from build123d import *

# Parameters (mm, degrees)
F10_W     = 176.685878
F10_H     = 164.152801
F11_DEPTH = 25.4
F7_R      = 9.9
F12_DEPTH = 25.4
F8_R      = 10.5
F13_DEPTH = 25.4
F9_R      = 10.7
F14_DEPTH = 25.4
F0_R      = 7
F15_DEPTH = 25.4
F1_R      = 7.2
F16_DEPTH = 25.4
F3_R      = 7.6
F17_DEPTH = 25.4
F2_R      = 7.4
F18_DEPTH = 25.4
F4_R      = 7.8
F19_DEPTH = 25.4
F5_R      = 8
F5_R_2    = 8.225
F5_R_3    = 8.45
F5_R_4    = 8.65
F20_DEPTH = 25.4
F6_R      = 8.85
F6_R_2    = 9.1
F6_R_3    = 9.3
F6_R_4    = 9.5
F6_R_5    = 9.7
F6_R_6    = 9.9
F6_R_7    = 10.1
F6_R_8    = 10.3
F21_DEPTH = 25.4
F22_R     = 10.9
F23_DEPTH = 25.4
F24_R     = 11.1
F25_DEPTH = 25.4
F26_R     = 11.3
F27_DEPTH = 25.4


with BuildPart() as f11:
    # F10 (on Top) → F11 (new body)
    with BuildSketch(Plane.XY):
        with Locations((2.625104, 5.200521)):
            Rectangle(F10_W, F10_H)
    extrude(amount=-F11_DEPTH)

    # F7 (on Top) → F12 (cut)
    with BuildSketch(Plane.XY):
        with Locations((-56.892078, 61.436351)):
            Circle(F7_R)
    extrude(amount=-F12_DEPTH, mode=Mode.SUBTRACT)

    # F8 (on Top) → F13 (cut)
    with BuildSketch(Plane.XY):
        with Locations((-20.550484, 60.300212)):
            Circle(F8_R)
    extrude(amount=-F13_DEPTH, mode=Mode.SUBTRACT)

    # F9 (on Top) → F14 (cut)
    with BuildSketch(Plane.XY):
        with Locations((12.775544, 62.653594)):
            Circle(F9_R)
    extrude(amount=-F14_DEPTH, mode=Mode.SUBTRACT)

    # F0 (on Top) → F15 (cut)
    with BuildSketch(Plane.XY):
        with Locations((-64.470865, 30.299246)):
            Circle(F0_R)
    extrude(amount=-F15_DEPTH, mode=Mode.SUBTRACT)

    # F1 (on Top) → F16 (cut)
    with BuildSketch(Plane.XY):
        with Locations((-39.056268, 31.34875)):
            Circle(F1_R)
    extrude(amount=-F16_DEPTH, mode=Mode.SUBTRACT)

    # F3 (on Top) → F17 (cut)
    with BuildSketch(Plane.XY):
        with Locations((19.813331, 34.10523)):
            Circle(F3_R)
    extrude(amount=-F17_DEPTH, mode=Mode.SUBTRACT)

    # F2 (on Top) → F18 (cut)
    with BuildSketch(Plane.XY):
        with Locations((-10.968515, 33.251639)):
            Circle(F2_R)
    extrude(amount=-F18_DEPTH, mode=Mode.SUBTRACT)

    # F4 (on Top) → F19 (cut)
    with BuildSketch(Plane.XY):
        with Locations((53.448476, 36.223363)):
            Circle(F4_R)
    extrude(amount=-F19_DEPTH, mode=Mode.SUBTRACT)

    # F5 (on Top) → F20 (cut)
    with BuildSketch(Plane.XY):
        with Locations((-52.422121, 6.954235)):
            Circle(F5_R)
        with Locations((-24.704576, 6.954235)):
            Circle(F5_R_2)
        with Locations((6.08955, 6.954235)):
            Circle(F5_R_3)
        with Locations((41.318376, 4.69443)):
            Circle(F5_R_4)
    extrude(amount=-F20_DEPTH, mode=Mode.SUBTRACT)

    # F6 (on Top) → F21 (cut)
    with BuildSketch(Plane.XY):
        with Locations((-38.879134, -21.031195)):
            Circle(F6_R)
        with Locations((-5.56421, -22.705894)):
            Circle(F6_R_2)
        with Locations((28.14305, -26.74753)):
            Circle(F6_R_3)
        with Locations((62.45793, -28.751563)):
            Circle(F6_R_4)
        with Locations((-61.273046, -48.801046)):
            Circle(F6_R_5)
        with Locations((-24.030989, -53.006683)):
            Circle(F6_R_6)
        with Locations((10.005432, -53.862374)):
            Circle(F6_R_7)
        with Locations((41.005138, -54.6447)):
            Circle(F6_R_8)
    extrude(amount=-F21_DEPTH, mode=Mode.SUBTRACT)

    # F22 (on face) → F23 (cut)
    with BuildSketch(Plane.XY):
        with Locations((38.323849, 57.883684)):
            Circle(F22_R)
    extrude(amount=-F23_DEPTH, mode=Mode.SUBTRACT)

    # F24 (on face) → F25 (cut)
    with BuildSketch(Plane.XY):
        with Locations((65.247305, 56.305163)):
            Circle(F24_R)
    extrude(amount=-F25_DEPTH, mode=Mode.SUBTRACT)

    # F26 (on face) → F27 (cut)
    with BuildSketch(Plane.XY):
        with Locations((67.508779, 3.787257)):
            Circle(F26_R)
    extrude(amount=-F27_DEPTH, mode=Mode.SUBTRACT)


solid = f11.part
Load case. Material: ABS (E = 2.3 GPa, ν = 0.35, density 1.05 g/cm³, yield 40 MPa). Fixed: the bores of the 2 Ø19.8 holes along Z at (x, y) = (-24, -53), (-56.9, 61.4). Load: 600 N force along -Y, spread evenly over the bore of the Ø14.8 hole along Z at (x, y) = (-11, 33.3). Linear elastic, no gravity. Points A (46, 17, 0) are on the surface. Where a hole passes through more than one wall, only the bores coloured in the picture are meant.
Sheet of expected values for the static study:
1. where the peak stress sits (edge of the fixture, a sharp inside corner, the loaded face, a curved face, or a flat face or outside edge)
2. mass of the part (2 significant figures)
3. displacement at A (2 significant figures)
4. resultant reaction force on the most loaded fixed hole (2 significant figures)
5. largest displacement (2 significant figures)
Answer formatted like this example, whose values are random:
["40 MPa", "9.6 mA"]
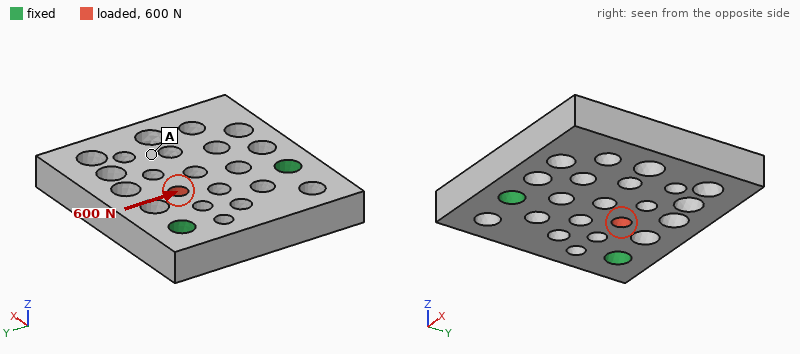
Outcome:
["the loaded face", "610 g", "11 µm", "330 N", "20 µm"]
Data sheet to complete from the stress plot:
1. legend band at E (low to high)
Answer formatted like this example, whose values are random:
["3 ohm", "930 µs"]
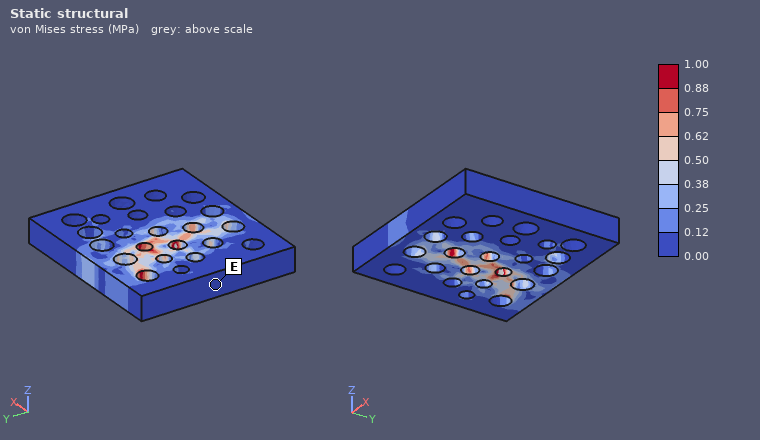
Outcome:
["0.00 to 0.12 MPa"]
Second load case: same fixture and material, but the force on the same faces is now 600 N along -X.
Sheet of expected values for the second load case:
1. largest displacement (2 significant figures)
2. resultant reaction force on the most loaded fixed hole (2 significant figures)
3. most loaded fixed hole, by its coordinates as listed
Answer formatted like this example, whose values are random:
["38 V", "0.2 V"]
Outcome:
["17 µm", "460 N", "(-56.9, 61.4)"]
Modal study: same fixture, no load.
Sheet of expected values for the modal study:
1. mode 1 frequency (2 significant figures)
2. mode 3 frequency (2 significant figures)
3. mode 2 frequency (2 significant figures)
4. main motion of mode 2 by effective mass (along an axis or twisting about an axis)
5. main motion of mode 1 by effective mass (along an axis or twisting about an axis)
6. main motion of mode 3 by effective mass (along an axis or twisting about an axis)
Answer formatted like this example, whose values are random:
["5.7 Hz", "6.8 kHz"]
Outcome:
["310 Hz", "1100 Hz", "600 Hz", "twisting about X", "along Z", "along Y"]
